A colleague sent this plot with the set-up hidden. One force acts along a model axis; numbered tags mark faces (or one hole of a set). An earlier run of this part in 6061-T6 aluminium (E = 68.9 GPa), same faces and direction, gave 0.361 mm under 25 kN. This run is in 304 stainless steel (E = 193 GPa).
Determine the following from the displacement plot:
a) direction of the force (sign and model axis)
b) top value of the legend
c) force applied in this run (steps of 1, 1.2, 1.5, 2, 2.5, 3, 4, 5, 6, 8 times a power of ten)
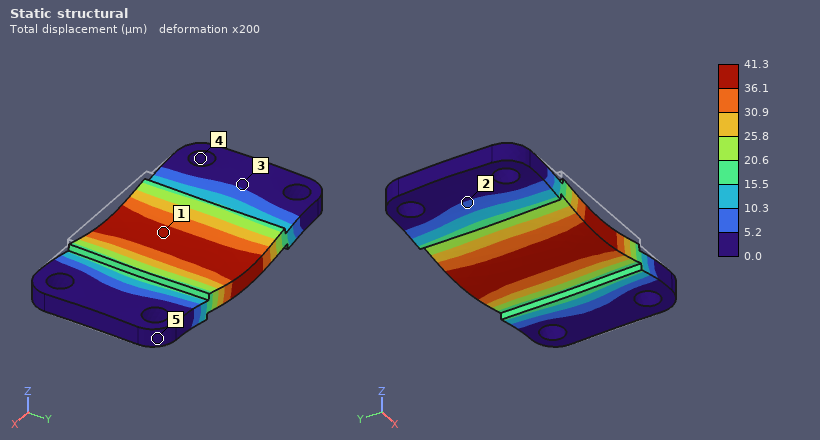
-Z
41.3 µm
8 kN
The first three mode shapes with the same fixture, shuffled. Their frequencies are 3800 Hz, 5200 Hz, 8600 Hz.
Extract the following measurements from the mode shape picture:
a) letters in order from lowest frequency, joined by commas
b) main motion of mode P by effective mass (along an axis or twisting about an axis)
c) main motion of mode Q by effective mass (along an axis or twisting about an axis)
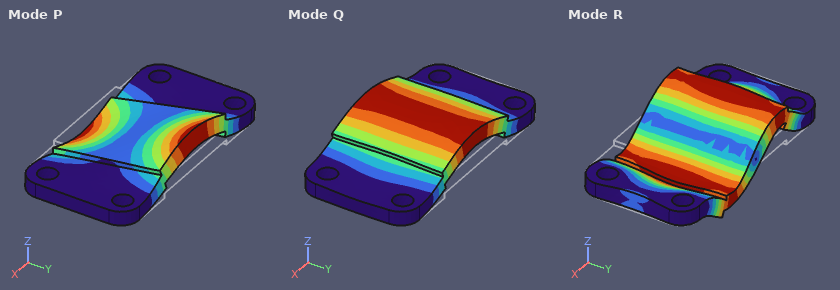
Q, P, R
twisting about X
along Z
